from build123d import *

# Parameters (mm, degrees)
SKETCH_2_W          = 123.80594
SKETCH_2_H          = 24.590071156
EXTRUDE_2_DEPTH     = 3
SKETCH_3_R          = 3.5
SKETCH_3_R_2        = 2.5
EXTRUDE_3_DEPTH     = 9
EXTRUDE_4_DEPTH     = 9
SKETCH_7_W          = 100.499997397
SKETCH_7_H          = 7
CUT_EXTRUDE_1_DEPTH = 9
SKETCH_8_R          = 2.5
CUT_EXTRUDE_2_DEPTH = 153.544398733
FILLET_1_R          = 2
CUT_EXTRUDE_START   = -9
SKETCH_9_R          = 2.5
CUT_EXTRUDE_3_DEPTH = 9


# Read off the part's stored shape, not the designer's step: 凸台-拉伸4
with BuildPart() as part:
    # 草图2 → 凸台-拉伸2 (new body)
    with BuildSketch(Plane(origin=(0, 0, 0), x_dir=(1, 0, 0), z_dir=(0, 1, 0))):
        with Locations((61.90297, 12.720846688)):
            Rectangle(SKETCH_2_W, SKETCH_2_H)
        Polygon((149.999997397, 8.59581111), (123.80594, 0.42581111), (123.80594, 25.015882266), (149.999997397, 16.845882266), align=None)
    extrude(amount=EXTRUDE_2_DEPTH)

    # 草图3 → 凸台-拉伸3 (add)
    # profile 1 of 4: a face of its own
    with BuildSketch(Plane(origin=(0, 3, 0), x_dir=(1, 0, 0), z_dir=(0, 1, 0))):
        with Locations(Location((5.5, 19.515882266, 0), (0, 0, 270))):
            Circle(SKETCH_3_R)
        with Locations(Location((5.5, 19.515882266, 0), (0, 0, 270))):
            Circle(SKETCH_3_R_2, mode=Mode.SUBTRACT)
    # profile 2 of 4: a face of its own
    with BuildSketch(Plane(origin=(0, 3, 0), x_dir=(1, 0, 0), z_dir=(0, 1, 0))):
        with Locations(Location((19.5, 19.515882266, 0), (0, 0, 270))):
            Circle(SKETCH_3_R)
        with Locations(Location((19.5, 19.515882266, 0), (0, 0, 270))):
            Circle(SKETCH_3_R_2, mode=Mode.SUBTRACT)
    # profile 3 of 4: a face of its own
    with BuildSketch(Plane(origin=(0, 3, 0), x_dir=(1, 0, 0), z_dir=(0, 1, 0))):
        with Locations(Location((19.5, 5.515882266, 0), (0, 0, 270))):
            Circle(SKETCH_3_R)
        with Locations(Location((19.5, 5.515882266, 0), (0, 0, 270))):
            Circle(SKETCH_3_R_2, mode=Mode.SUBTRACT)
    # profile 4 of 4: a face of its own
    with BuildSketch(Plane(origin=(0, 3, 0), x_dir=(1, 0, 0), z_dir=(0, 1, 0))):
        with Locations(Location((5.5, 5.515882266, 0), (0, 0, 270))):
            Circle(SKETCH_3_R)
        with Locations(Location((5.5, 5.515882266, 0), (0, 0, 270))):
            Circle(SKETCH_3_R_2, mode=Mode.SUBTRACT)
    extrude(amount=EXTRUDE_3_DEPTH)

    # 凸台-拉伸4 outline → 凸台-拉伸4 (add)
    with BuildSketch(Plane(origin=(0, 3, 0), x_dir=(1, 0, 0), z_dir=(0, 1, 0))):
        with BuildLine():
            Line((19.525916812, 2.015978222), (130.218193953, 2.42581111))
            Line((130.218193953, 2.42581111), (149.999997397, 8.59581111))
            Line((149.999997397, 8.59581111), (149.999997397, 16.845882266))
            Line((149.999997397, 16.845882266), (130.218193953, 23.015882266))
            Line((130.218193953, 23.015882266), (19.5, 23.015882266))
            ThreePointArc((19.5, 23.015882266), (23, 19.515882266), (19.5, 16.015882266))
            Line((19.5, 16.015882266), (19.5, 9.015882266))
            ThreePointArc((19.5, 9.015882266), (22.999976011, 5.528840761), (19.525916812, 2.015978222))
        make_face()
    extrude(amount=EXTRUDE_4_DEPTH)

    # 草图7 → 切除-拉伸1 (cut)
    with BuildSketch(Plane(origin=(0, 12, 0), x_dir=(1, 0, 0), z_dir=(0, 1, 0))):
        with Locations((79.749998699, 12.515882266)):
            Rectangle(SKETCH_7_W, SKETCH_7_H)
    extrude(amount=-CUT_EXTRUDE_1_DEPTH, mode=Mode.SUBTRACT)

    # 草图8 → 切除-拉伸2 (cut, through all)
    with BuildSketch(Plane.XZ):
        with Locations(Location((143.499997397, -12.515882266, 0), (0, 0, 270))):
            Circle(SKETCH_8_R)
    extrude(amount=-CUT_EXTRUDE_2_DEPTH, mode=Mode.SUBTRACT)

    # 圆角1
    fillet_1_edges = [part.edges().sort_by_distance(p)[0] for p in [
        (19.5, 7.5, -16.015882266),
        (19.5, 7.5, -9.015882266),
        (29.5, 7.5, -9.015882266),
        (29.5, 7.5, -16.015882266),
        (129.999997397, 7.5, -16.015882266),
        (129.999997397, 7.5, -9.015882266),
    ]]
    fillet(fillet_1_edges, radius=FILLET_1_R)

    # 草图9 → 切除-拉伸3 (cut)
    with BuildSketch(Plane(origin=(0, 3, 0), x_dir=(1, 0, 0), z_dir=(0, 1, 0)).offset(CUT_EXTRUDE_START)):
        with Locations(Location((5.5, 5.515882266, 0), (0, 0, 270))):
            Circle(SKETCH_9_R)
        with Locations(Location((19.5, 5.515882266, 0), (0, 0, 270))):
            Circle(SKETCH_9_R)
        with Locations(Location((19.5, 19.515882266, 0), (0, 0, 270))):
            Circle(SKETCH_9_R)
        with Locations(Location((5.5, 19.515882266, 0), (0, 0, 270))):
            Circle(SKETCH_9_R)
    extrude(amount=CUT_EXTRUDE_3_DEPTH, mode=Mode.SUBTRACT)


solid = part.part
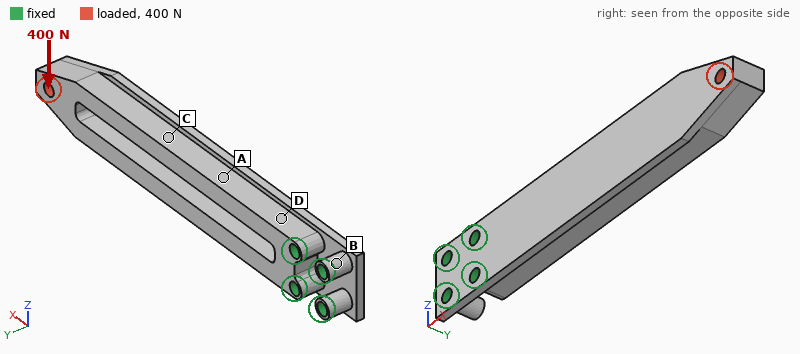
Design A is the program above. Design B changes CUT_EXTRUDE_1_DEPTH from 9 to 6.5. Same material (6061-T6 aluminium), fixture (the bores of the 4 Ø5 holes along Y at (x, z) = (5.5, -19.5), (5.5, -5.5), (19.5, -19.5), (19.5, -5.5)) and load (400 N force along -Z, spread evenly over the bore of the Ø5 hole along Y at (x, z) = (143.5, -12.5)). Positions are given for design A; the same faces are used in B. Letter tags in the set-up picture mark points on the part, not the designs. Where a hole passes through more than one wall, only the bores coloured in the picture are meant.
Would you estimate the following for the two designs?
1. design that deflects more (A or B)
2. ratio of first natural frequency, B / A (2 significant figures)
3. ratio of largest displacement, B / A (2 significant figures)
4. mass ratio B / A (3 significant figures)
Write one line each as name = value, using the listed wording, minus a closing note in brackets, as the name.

design that deflects more = A
ratio of first natural frequency, B / A = 0.98
ratio of largest displacement, B / A = 0.92
mass ratio B / A = 1.06
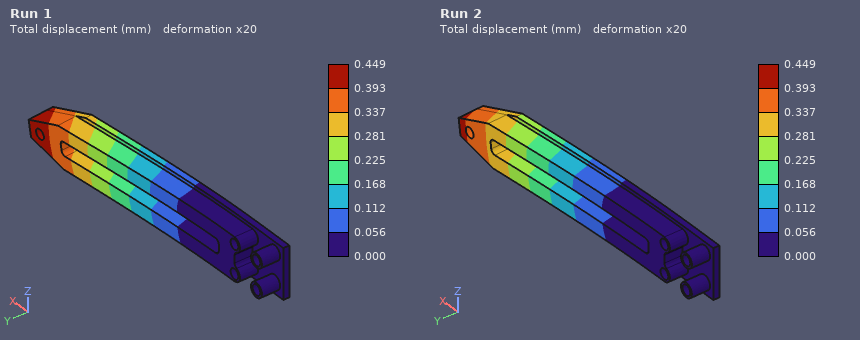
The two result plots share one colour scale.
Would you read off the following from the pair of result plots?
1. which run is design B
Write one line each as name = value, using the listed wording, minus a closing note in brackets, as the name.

which run is design B = Run 2
